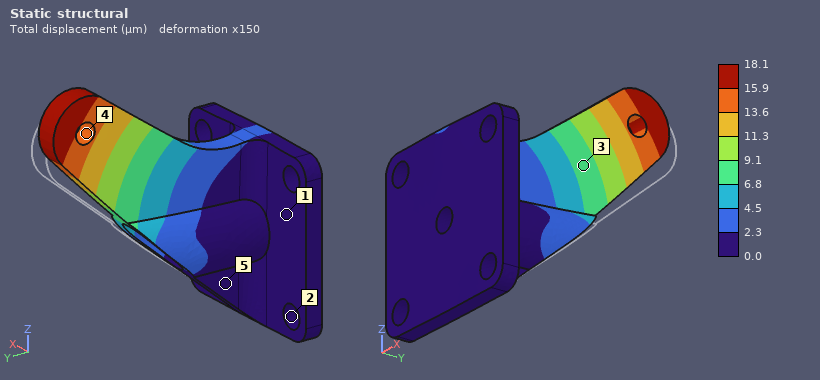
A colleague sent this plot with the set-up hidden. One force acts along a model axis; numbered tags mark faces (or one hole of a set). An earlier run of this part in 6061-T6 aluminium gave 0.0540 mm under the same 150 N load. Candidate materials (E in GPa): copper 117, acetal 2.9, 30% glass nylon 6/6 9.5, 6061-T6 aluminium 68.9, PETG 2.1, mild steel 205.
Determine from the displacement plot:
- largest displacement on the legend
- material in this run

18.1 µm
mild steel
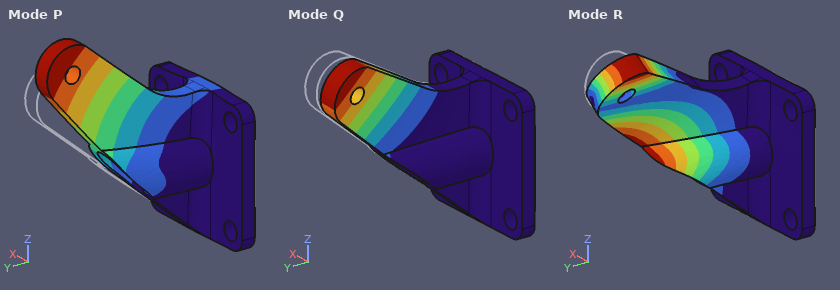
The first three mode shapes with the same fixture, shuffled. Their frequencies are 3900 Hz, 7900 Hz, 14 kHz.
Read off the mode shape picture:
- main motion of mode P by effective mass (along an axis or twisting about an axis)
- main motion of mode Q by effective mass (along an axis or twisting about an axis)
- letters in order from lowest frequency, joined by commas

along Z
along X
Q, P, R
